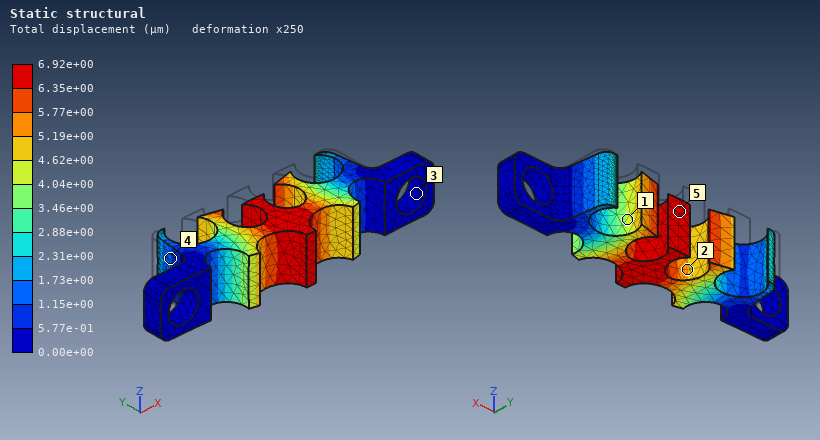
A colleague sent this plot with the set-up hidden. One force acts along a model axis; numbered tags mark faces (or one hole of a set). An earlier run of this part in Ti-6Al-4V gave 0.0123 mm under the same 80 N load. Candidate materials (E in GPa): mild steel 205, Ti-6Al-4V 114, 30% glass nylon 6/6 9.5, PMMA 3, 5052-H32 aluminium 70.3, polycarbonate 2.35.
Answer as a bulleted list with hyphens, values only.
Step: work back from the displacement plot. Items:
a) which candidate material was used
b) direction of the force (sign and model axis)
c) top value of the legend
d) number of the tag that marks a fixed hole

- mild steel
- -Y
- 6.92e+00 µm
- 3
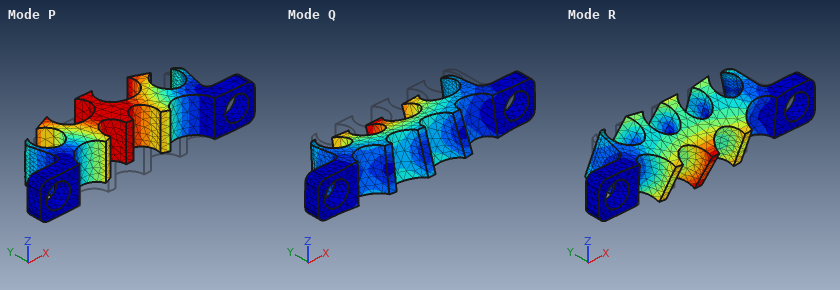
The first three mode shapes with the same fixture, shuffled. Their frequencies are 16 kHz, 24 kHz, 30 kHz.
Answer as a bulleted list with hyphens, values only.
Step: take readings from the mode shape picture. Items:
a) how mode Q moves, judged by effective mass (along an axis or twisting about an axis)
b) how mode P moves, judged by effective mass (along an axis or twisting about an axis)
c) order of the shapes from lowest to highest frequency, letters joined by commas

- along Z
- along Y
- P, Q, R
